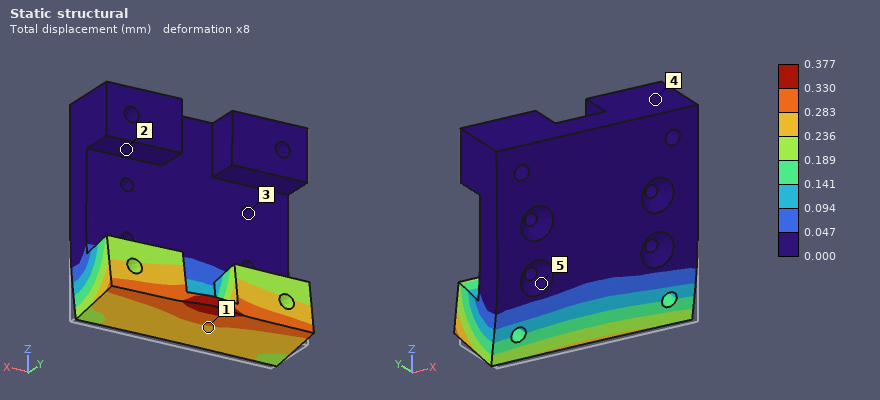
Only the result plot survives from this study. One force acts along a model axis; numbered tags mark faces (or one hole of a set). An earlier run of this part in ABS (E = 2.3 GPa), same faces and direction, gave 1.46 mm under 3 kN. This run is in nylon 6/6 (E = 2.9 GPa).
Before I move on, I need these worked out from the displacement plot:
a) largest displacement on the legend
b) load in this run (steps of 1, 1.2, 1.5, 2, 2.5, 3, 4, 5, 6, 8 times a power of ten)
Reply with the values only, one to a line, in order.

0.377 mm
1 kN
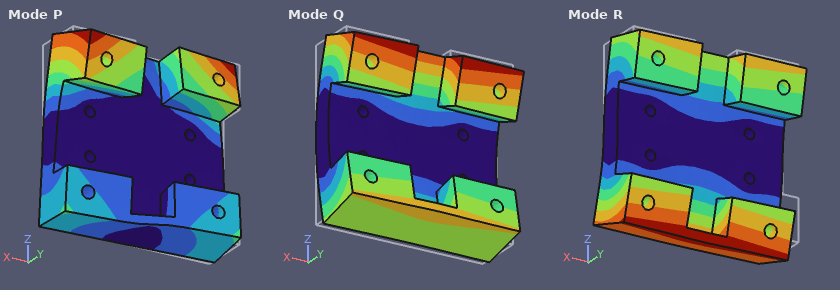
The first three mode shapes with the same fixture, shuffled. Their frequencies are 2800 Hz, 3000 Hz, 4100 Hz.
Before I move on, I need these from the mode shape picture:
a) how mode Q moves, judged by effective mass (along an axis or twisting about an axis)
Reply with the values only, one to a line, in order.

along Y
